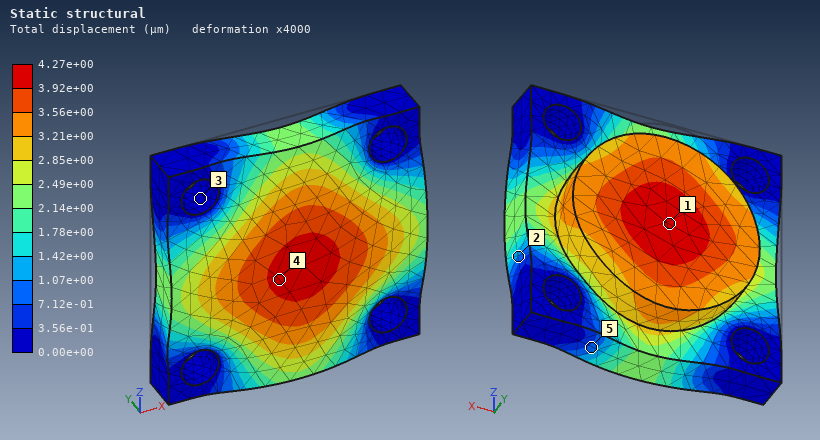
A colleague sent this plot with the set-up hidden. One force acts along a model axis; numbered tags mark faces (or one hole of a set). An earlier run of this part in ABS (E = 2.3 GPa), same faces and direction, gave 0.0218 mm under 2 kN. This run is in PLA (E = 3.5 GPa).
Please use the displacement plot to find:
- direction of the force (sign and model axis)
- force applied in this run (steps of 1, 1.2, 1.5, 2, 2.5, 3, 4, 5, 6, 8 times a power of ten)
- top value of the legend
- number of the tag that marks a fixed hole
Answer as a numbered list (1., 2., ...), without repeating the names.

1. -Y
2. 600 N
3. 4.27e+00 µm
4. 3
